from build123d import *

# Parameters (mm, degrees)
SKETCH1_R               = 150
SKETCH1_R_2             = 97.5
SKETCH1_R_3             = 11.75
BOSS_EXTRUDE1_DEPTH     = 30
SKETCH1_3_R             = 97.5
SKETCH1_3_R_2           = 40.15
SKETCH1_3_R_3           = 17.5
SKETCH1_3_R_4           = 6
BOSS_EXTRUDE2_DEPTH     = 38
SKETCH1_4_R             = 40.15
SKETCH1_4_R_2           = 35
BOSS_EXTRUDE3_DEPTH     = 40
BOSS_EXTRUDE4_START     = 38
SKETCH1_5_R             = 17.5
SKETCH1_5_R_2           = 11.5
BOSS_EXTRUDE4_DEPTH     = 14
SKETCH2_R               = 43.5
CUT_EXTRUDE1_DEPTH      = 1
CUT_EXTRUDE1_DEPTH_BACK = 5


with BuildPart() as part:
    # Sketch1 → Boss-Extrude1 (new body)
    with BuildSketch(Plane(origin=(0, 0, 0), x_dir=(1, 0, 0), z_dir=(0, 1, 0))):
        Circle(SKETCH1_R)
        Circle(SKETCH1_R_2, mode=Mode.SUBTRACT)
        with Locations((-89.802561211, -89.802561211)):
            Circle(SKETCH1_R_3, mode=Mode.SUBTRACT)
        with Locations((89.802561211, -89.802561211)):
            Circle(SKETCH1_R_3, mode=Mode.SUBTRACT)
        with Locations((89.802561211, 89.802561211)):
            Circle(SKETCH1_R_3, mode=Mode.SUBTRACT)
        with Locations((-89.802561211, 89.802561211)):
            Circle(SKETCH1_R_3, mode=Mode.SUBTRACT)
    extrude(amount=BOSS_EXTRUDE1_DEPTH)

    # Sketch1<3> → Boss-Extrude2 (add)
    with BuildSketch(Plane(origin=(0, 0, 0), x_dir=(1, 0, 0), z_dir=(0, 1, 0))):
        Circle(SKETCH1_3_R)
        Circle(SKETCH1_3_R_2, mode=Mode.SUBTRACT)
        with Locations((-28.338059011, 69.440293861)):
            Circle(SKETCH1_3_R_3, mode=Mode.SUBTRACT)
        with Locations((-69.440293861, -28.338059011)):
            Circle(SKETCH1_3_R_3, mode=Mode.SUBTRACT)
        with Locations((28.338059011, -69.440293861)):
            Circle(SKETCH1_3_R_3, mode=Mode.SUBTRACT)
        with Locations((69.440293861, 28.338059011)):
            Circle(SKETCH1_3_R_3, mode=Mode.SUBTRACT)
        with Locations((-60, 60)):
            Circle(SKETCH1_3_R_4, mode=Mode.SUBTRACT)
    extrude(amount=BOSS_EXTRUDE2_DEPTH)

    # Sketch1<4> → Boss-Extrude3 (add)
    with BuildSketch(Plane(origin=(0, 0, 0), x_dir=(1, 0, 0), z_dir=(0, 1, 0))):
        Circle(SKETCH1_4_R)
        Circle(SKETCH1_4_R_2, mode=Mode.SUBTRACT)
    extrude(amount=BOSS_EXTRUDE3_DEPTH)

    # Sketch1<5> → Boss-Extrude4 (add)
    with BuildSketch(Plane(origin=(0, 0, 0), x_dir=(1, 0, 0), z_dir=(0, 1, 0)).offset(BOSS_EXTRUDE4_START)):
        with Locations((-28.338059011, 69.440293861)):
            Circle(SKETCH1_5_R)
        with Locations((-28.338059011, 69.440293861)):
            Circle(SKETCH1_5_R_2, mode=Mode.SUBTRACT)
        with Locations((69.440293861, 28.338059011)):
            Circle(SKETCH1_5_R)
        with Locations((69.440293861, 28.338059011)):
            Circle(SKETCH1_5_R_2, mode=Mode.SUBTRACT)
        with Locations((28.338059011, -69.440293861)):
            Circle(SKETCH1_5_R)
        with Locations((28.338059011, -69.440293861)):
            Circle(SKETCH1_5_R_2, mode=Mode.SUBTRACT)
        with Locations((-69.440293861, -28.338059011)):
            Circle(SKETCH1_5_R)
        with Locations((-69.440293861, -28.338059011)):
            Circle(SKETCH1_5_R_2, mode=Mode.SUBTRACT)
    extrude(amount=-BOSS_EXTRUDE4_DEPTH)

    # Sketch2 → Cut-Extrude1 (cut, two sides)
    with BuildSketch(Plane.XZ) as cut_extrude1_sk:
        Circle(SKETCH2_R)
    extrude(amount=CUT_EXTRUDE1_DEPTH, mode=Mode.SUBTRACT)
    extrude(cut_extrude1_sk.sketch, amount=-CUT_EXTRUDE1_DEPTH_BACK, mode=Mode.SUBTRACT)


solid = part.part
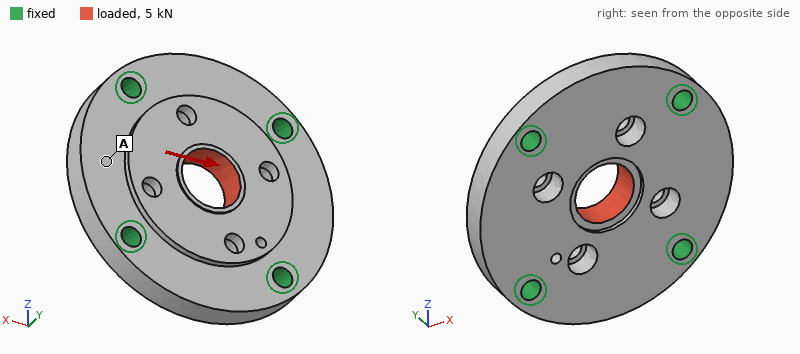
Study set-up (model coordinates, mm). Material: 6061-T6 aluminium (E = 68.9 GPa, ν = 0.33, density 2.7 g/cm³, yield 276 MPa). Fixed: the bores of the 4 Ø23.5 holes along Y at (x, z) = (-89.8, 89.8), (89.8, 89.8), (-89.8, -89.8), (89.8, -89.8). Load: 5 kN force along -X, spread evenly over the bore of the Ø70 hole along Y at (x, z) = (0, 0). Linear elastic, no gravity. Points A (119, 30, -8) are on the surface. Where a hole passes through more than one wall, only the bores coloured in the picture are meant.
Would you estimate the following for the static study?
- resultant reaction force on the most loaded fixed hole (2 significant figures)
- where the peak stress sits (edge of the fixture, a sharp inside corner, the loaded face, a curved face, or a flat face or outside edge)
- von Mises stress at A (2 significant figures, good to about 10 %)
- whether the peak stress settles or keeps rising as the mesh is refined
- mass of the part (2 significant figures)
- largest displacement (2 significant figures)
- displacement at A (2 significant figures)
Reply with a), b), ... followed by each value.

a) 1.4 kN
b) edge of the fixture
c) 0.32 MPa
d) keeps rising
e) 5.5 kg
f) 1.6 µm
g) 0.91 µm
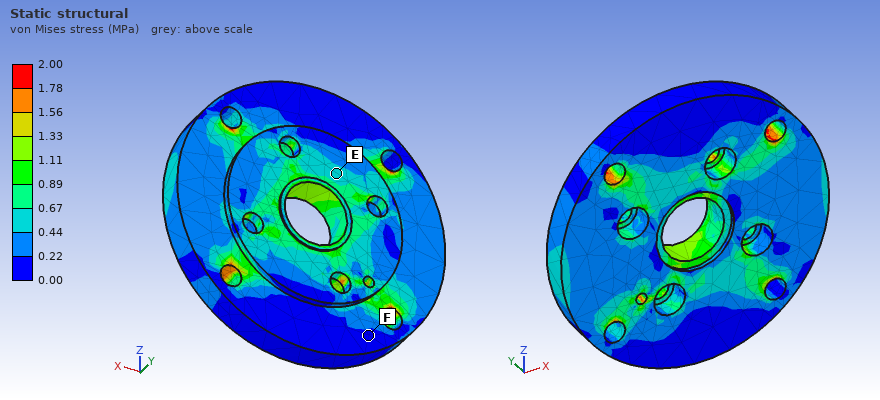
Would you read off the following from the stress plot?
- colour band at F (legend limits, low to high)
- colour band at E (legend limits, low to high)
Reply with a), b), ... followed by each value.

a) 0.00 to 0.22 MPa
b) 0.44 to 0.67 MPa
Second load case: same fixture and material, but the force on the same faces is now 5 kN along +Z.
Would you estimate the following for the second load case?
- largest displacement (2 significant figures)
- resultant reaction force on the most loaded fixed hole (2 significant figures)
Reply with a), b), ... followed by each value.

a) 1.6 µm
b) 1.4 kN
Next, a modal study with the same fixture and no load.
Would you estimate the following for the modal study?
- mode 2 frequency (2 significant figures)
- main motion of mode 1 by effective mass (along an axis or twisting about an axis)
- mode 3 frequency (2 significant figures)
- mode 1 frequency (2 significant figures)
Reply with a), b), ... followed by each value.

a) 3700 Hz
b) along Y
c) 3800 Hz
d) 3400 Hz
